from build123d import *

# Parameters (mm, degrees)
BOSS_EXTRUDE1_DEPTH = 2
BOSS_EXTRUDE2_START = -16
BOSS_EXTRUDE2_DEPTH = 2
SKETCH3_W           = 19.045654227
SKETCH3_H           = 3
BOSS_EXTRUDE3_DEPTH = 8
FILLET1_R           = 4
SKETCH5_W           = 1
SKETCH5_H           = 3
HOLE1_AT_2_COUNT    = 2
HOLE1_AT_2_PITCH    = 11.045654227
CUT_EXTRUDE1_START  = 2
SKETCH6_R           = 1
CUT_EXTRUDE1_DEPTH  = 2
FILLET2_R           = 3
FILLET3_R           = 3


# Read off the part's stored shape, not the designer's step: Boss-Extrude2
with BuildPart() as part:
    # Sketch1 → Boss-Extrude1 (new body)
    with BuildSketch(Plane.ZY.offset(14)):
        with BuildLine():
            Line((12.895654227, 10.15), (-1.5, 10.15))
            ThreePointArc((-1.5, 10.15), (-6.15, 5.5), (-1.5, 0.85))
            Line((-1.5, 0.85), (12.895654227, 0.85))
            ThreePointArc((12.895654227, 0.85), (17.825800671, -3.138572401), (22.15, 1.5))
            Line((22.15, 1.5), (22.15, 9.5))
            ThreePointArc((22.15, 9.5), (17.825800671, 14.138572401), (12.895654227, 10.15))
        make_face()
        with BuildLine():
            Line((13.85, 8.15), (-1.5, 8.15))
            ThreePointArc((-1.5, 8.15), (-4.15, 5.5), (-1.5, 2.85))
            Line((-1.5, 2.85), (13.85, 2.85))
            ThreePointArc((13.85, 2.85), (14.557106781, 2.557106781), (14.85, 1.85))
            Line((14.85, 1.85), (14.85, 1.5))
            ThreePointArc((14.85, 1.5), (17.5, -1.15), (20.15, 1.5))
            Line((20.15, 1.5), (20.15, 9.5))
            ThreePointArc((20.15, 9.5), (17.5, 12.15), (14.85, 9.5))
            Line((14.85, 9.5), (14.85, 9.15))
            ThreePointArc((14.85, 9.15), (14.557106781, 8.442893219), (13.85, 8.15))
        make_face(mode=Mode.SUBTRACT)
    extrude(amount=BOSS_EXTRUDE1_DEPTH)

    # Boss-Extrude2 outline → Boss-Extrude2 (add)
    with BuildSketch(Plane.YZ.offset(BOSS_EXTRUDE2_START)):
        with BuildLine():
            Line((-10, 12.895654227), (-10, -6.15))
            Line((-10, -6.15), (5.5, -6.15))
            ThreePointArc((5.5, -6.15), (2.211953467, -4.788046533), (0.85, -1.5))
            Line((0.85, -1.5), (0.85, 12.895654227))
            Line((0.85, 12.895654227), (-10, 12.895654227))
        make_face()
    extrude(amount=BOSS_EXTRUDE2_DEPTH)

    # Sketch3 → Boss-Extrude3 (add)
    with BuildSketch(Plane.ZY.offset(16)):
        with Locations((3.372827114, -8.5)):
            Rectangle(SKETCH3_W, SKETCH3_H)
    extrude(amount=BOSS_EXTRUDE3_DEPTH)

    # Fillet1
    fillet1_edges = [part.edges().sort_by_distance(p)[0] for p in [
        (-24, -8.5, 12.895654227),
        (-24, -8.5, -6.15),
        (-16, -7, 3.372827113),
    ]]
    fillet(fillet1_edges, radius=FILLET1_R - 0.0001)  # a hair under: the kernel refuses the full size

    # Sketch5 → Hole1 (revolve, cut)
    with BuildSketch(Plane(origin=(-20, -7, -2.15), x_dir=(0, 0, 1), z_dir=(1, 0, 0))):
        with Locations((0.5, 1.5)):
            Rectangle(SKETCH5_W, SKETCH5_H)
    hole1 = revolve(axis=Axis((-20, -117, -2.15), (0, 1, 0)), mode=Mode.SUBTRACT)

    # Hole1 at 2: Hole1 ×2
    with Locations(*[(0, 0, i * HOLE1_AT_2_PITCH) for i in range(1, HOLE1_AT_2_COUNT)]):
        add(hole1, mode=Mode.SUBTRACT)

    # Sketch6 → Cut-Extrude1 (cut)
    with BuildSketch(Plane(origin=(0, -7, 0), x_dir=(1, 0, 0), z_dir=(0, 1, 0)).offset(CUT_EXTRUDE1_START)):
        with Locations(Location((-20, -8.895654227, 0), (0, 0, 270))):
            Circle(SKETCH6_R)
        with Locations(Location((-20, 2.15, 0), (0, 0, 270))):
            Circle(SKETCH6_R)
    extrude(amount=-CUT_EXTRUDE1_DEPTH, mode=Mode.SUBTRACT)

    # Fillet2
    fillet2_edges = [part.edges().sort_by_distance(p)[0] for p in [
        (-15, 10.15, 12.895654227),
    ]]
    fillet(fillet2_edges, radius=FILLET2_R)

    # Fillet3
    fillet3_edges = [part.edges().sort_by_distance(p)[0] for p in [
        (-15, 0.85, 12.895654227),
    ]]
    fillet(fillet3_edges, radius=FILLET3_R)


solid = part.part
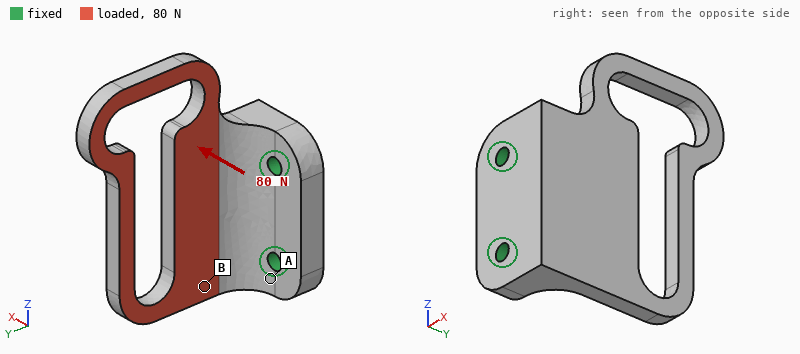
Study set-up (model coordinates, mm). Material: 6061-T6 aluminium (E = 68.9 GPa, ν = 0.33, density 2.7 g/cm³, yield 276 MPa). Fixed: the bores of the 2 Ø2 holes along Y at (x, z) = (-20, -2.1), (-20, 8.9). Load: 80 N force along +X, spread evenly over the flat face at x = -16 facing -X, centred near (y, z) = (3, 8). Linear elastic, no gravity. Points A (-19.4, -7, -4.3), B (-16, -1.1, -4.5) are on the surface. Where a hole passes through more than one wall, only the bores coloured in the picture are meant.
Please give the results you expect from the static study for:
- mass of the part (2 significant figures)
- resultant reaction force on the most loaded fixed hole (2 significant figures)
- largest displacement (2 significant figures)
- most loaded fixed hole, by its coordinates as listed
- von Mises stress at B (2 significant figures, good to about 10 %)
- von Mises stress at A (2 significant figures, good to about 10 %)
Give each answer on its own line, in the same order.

3.3 g
67 N
0.37 mm
(-20, 8.9)
36 MPa
17 MPa
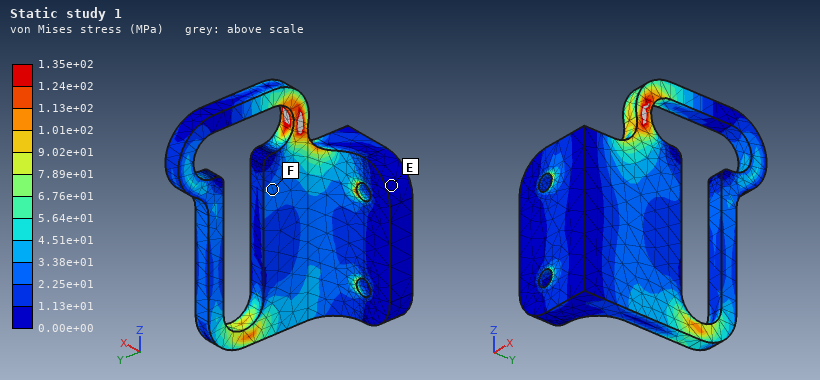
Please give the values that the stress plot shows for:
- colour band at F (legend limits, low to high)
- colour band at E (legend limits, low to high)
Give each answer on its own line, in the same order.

2.25e+01 to 3.38e+01 MPa
0.00e+00 to 1.13e+01 MPa
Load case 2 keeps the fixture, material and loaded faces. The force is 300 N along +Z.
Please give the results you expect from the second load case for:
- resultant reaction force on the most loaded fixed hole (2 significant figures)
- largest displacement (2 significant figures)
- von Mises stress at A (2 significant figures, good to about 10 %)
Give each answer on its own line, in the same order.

320 N
0.14 mm
38 MPa
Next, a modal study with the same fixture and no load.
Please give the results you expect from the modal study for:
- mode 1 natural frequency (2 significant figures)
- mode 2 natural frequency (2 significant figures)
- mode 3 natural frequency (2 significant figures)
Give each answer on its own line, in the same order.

2700 Hz
7100 Hz
7600 Hz
